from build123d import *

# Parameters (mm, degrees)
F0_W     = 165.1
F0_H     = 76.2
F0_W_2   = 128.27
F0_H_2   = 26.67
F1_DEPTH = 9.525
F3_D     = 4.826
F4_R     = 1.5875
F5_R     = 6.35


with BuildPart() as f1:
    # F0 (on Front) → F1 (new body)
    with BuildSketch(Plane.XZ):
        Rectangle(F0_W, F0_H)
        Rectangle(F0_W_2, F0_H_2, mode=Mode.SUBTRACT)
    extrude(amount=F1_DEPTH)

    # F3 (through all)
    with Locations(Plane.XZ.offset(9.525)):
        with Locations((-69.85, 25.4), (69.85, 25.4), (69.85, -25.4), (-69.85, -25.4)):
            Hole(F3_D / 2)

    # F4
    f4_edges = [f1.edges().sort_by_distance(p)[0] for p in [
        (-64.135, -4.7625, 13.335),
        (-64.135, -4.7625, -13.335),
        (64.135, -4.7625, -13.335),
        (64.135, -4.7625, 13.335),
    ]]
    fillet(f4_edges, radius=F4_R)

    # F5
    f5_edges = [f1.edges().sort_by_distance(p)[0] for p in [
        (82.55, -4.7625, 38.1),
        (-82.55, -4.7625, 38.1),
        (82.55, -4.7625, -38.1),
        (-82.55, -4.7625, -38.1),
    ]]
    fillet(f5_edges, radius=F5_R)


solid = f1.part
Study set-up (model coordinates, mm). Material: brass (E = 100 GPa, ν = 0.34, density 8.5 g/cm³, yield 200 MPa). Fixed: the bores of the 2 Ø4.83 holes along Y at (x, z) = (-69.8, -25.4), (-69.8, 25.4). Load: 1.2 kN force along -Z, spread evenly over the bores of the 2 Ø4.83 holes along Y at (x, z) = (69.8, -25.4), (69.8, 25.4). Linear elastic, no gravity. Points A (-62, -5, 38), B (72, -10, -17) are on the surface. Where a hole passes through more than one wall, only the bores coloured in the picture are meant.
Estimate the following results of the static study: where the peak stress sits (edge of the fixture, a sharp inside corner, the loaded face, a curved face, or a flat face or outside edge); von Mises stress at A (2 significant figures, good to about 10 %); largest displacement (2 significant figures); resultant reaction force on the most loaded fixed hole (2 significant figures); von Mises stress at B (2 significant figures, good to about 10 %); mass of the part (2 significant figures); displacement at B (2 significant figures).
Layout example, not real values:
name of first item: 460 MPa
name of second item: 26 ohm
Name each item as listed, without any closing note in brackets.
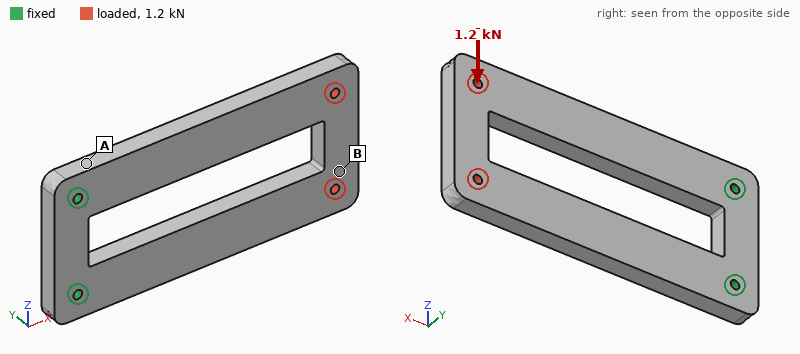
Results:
where the peak stress sits: a curved face
von Mises stress at A: 39 MPa
largest displacement: 0.22 mm
resultant reaction force on the most loaded fixed hole: 2.8 kN
von Mises stress at B: 14 MPa
mass of the part: 730 g
displacement at B: 0.21 mm
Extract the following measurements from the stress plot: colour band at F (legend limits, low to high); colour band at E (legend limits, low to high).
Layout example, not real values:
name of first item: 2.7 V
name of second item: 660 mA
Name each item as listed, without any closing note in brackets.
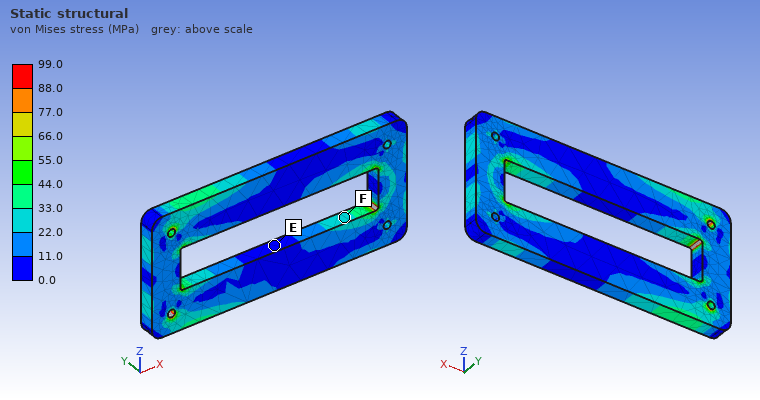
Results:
colour band at F: 22.0 to 33.0 MPa
colour band at E: 0.0 to 11.0 MPa
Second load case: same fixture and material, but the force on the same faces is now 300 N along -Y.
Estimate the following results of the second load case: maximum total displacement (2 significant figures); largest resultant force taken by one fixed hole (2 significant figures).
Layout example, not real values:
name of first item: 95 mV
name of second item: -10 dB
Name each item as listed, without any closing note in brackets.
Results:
maximum total displacement: 0.89 mm
largest resultant force taken by one fixed hole: 150 N
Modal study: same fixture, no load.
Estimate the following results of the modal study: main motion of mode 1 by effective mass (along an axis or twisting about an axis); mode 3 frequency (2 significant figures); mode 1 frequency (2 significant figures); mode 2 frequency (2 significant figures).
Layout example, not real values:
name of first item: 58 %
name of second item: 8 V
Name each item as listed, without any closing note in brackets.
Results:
main motion of mode 1 by effective mass: along Y
mode 3 frequency: 720 Hz
mode 1 frequency: 200 Hz
mode 2 frequency: 700 Hz
